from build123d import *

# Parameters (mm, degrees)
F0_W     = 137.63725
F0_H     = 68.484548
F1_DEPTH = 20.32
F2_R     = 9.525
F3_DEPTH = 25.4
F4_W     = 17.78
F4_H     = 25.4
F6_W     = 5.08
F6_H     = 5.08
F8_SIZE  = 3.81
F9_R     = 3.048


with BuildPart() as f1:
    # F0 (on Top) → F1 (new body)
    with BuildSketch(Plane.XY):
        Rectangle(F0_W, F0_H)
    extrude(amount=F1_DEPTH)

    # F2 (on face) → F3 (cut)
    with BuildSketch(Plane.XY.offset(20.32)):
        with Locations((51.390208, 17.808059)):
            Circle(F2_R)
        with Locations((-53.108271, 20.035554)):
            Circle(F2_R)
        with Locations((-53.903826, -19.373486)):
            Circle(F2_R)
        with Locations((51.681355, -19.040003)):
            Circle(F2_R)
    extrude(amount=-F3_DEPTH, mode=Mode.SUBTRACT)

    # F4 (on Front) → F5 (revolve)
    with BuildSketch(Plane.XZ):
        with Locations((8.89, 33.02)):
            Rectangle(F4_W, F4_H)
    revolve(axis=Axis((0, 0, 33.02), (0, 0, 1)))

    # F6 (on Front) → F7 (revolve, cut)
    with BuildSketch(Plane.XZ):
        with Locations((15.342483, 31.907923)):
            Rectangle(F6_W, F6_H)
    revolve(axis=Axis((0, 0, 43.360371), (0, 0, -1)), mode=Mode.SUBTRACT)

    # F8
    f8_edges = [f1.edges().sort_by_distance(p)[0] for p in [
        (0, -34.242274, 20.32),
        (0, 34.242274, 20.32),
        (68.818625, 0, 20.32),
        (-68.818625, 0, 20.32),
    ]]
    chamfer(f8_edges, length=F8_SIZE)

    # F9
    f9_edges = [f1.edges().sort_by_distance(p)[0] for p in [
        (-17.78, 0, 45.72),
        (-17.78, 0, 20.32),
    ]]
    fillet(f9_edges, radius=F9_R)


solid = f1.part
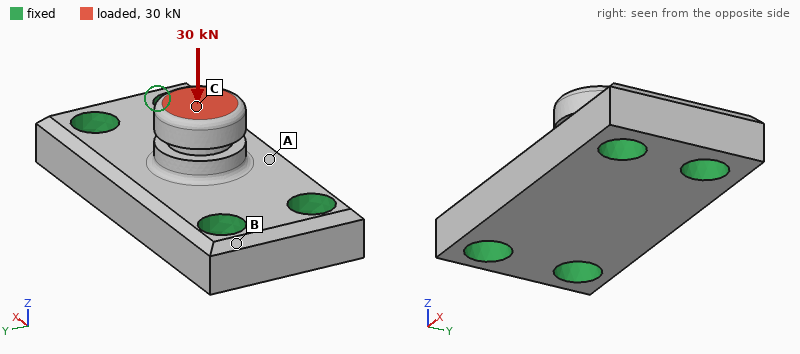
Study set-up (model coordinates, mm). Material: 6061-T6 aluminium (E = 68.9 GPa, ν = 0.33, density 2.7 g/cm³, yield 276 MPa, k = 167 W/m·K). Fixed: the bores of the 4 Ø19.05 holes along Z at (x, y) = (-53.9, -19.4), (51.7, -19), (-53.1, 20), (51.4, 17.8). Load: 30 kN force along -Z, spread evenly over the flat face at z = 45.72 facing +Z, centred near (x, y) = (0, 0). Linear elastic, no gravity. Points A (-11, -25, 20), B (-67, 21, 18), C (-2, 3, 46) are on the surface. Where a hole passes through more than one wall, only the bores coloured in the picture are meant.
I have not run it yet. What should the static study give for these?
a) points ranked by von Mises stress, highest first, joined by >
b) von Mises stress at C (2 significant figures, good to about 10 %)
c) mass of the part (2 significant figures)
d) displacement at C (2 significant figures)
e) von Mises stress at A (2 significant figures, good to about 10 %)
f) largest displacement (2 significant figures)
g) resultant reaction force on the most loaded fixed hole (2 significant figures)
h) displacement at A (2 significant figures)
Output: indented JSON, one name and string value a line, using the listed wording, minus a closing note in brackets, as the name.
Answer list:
{
  "points ranked by von Mises stress, highest first, joined by >": "C > A > B",
  "von Mises stress at C": "50 MPa",
  "mass of the part": "510 g",
  "displacement at C": "58 µm",
  "von Mises stress at A": "30 MPa",
  "largest displacement": "59 µm",
  "resultant reaction force on the most loaded fixed hole": "8.1 kN",
  "displacement at A": "36 µm"
}
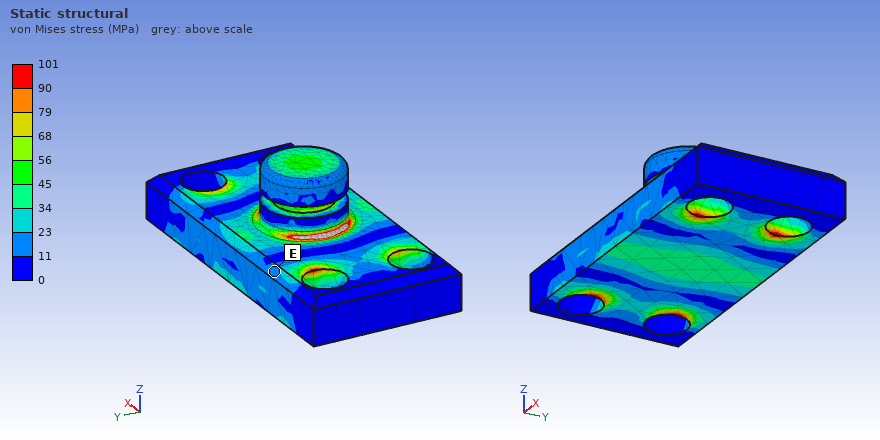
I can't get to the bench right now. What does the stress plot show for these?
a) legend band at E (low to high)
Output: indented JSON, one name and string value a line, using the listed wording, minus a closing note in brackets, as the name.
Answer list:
{
  "legend band at E": "11 to 23 MPa"
}
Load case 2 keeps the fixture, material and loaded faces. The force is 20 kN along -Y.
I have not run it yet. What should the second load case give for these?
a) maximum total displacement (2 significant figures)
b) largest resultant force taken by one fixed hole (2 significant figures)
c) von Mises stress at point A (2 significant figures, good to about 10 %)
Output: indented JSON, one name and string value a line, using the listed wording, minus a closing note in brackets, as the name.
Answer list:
{
  "maximum total displacement": "0.18 mm",
  "largest resultant force taken by one fixed hole": "10 kN",
  "von Mises stress at point A": "34 MPa"
}
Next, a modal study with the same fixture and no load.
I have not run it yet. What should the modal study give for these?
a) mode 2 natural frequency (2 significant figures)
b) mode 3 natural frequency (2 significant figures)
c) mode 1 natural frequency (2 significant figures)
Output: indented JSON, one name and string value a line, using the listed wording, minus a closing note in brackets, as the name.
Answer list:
{
  "mode 2 natural frequency": "8900 Hz",
  "mode 3 natural frequency": "13 kHz",
  "mode 1 natural frequency": "8800 Hz"
}
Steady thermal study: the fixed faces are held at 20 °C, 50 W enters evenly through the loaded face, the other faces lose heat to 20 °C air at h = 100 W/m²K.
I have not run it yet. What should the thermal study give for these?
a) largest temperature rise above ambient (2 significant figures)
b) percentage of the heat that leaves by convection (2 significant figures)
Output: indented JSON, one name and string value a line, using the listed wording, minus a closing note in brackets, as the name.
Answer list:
{
  "largest temperature rise above ambient": "16 K",
  "percentage of the heat that leaves by convection": "13 %"
}
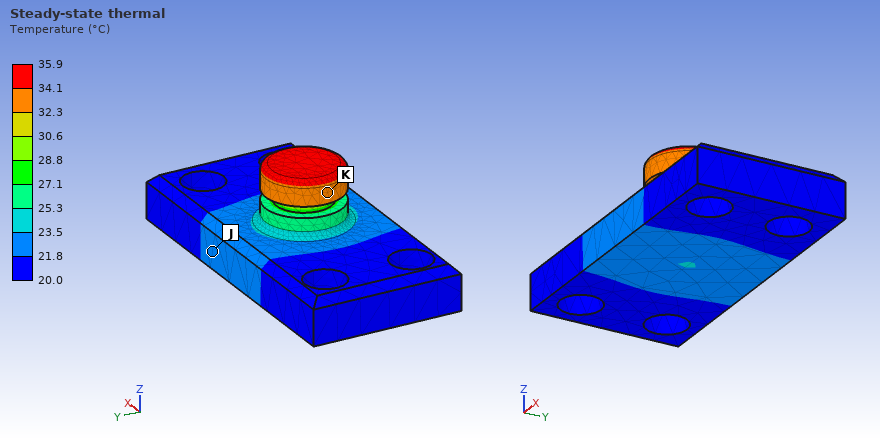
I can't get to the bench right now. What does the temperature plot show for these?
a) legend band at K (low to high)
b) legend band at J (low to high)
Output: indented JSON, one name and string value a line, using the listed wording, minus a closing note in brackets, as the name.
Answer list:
{
  "legend band at K": "32.3 to 34.1 °C",
  "legend band at J": "21.8 to 23.5 °C"
}
